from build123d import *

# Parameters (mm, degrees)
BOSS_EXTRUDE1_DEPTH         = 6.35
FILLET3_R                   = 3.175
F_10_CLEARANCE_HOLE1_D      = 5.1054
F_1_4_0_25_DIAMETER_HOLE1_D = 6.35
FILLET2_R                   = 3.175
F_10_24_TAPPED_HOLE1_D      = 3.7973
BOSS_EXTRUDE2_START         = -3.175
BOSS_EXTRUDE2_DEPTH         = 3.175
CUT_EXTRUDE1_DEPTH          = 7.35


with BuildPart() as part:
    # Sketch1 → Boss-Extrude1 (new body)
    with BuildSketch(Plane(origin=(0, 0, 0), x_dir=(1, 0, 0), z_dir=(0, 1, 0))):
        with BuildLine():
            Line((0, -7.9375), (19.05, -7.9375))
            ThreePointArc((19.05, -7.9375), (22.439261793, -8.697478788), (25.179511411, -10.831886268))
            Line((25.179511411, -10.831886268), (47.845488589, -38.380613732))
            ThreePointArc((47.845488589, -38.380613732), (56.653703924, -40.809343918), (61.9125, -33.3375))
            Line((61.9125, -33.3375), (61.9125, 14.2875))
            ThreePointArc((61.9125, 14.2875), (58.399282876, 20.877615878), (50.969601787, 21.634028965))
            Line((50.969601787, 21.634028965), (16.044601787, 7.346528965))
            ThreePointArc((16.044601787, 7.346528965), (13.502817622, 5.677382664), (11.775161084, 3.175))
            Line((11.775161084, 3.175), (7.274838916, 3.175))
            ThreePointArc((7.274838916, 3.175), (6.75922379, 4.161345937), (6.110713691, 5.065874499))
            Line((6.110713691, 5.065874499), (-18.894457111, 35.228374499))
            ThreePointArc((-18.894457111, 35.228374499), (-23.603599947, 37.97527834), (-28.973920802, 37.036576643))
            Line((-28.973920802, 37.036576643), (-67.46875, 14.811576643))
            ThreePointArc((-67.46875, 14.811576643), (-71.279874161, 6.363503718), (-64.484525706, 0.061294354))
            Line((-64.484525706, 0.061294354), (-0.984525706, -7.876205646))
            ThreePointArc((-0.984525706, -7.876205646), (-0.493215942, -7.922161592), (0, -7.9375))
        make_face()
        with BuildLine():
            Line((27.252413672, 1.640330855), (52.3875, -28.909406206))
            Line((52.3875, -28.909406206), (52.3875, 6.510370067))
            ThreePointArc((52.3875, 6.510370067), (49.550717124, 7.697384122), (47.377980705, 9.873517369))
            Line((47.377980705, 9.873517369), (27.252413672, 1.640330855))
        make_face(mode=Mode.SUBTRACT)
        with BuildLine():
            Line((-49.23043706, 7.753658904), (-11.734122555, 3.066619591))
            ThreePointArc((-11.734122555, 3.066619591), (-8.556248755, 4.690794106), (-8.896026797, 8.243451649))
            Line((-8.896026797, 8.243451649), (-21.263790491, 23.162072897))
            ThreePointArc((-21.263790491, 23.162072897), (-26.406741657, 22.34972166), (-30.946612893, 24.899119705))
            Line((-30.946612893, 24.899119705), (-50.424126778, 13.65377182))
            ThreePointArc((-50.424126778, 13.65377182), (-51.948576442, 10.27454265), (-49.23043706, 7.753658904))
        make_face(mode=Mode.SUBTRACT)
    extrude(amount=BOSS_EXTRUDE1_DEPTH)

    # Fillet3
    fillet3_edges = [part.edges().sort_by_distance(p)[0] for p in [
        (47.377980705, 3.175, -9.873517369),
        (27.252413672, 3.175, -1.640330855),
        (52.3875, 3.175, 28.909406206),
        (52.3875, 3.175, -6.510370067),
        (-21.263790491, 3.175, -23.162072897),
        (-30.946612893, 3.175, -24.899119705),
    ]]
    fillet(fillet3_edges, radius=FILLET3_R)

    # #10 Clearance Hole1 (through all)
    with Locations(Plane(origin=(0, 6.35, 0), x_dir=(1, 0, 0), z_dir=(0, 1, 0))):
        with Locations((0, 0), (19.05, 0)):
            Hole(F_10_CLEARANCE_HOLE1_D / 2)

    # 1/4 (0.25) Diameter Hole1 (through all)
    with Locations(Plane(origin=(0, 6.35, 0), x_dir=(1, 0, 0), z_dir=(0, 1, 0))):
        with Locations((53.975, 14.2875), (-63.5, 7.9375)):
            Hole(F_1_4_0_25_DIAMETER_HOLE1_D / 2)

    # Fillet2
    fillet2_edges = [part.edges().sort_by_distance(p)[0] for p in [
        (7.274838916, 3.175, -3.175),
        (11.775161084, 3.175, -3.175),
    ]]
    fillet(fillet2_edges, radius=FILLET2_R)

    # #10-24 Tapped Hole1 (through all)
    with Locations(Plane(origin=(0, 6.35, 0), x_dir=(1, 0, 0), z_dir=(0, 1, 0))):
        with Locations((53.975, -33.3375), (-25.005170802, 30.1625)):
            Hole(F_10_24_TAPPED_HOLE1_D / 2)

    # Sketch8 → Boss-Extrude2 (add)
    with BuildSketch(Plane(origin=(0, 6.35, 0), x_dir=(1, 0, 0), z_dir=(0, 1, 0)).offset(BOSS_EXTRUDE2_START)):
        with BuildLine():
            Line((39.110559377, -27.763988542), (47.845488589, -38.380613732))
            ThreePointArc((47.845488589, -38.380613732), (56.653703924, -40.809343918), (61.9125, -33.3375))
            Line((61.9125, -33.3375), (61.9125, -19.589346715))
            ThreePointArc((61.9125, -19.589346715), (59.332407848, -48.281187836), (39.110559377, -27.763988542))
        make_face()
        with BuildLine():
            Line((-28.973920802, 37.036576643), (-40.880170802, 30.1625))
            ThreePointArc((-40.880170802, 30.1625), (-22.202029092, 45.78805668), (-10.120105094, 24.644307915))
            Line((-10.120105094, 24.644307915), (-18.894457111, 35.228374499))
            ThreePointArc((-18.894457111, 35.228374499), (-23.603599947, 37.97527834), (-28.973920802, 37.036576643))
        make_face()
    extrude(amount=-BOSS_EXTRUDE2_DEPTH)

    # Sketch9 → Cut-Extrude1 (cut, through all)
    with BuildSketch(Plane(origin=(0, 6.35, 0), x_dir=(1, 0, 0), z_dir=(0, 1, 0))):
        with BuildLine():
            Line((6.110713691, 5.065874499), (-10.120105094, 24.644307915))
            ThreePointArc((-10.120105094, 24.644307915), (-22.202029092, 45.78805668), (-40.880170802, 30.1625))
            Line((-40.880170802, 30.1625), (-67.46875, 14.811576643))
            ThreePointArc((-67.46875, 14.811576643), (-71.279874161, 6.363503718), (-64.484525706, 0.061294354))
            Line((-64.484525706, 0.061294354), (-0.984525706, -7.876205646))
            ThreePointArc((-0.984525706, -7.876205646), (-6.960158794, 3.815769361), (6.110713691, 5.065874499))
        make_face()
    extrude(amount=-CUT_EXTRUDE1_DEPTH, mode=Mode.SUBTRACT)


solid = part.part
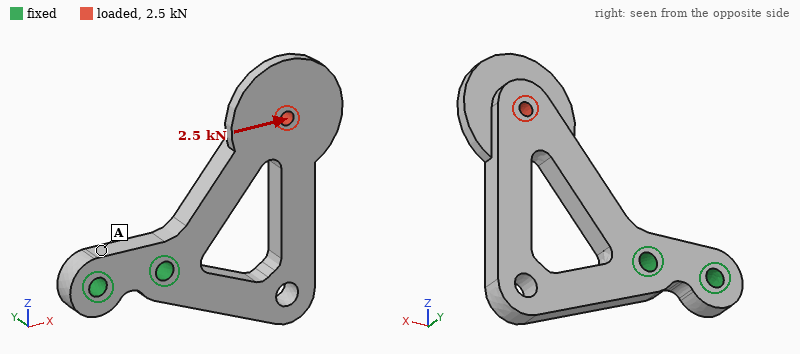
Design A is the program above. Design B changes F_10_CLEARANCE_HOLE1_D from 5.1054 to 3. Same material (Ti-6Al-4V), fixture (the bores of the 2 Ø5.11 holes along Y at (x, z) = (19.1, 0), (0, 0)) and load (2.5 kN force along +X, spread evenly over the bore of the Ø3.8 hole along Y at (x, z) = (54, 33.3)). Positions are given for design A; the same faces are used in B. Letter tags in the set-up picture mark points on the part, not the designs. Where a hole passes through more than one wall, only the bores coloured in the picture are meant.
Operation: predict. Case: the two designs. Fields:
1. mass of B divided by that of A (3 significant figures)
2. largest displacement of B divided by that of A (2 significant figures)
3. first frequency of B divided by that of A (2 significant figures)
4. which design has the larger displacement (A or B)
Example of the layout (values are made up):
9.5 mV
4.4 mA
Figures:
1.01
1.2
0.95
B
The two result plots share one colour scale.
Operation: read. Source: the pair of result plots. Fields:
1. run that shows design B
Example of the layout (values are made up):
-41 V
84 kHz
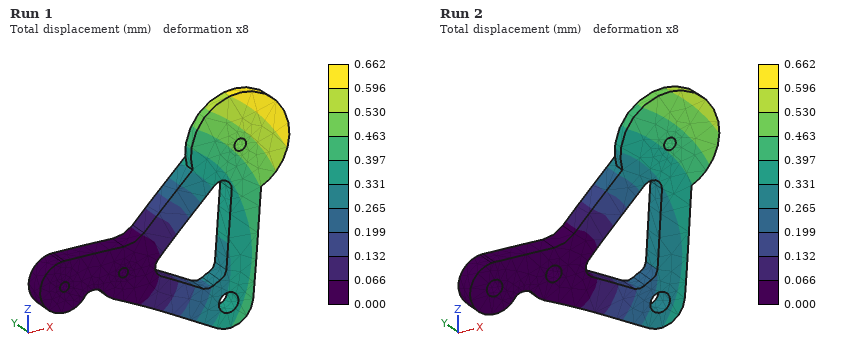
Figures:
Run 1
